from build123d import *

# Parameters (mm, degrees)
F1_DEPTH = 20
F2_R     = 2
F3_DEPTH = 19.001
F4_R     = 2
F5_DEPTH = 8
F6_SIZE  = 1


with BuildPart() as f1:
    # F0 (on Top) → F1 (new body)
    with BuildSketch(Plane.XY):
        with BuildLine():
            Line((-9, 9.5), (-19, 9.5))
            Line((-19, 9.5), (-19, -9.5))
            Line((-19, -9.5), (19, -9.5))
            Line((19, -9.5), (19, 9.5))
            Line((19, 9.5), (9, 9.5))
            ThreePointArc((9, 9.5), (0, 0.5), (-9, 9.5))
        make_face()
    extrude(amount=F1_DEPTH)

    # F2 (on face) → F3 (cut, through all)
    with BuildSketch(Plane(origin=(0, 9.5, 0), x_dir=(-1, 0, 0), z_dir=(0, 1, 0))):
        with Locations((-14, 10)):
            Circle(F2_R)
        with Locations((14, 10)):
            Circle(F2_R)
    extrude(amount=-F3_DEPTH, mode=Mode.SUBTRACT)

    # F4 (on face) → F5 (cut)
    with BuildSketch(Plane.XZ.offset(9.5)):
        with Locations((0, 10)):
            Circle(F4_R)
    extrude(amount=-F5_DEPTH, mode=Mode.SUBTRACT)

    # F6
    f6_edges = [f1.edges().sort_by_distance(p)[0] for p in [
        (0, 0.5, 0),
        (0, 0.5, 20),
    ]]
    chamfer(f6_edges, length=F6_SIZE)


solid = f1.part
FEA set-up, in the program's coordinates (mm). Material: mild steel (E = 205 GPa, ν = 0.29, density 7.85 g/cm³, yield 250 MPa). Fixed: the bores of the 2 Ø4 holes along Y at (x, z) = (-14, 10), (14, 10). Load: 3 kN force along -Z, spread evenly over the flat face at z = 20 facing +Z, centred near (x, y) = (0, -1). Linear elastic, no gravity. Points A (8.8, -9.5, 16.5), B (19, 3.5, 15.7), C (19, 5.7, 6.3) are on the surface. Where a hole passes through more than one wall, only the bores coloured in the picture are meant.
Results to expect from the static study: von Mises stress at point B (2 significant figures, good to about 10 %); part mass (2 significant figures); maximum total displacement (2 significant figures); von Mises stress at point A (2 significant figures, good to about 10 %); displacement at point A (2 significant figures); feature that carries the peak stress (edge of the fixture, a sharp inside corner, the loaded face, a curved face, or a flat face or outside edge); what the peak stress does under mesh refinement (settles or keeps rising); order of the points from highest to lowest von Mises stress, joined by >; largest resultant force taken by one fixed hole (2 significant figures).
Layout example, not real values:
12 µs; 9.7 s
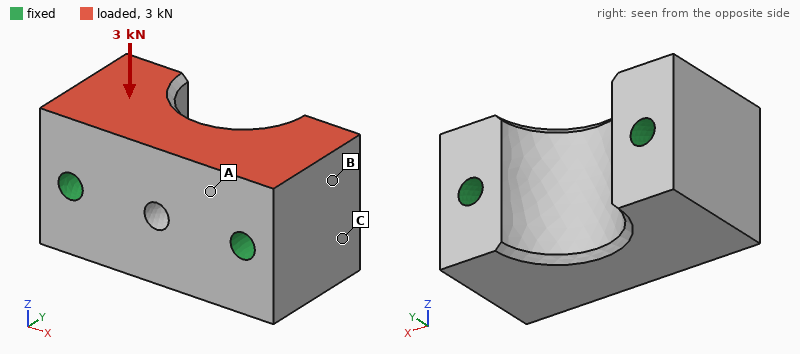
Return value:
4.0 MPa; 89 g; 0.78 µm; 6.7 MPa; 0.44 µm; edge of the fixture; keeps rising; A > B > C; 1.5 kN
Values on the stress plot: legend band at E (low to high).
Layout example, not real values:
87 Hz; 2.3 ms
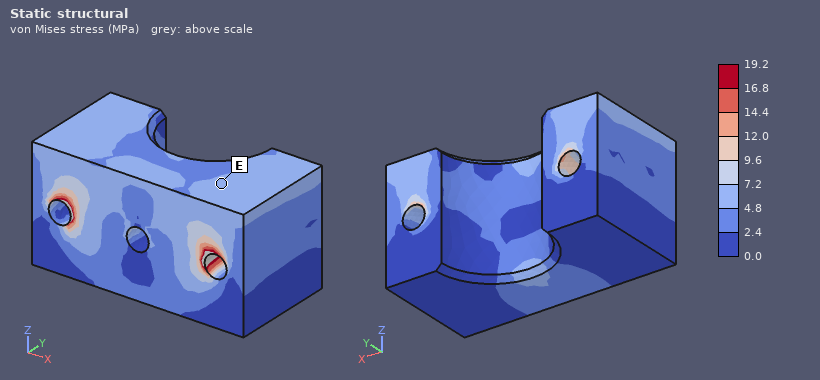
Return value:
4.8 to 7.2 MPa
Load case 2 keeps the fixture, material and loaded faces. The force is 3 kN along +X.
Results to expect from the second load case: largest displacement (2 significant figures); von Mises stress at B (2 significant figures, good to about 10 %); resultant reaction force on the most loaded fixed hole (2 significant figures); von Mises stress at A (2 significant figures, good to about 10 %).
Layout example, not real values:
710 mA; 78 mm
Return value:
1.6 µm; 9.9 MPa; 1.7 kN; 12 MPa
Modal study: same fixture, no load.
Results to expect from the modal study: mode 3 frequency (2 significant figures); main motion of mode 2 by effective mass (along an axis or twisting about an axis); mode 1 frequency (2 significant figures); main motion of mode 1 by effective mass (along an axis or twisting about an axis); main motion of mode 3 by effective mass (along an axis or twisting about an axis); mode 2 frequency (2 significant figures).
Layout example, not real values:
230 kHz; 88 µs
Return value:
54 kHz; along Y; 41 kHz; along Z; twisting about X; 47 kHz
